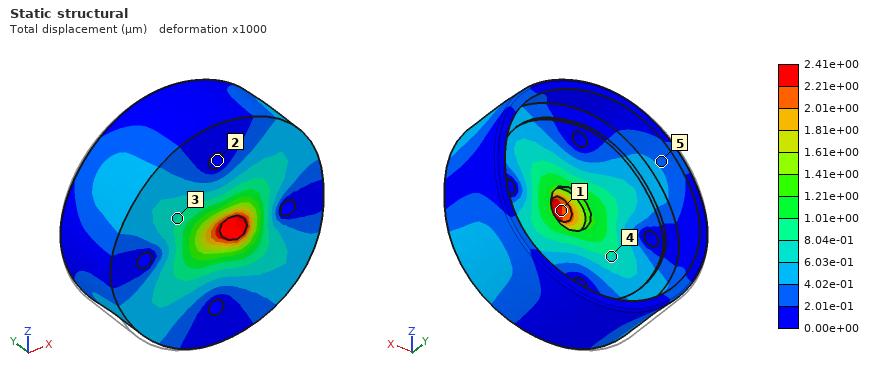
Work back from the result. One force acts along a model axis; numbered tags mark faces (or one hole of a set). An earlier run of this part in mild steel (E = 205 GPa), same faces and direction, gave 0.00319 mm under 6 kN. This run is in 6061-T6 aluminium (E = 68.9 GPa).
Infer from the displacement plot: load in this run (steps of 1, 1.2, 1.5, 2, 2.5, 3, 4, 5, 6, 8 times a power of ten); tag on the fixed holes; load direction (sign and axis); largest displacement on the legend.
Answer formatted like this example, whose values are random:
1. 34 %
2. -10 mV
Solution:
1. 1.5 kN
2. 2
3. +X
4. 2.41e+00 µm
